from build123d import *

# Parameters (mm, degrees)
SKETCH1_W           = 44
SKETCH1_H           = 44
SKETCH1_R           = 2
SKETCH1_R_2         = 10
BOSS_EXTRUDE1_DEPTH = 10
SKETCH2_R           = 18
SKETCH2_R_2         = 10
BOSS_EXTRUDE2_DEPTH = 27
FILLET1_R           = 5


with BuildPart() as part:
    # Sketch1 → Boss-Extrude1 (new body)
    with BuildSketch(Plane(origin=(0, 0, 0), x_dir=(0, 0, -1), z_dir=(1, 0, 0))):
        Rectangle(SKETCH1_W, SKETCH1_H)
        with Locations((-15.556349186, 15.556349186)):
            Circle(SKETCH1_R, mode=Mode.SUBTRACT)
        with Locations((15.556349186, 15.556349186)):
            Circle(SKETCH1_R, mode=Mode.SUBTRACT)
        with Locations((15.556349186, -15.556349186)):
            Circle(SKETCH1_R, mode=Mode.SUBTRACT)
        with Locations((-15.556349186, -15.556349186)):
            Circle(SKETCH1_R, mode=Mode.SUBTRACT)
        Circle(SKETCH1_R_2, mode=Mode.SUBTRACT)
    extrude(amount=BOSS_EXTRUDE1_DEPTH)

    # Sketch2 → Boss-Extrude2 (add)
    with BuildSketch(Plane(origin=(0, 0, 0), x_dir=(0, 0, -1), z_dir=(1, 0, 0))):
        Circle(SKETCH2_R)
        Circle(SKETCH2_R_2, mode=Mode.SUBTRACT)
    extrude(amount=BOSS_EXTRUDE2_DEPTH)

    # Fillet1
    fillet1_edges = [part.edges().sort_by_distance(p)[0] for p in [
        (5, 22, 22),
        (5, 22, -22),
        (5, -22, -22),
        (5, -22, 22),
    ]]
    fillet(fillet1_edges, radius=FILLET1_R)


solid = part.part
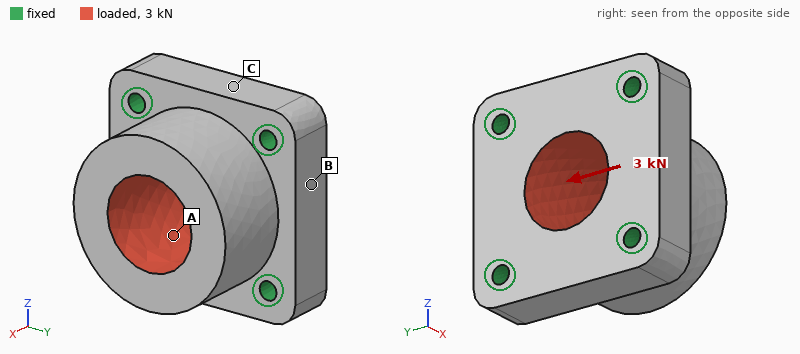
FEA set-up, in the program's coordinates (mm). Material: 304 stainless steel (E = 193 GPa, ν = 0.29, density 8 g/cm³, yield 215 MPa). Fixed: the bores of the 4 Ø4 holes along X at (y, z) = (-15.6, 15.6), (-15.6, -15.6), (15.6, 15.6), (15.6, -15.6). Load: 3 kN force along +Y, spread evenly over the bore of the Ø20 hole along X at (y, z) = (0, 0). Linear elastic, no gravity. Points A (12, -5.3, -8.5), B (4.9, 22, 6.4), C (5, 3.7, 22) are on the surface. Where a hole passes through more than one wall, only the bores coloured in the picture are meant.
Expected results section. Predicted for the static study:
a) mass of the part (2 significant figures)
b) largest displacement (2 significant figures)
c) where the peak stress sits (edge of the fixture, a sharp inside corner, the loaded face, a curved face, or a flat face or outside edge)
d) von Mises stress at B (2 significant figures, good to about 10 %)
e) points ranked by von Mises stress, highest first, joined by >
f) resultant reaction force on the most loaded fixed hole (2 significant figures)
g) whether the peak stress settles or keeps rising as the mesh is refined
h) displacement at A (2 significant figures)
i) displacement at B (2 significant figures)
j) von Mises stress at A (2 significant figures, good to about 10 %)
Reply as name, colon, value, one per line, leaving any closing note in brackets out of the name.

mass of the part: 220 g
largest displacement: 1.7 µm
where the peak stress sits: edge of the fixture
von Mises stress at B: 4.5 MPa
points ranked by von Mises stress, highest first, joined by >: A > B > C
resultant reaction force on the most loaded fixed hole: 870 N
whether the peak stress settles or keeps rising as the mesh is refined: keeps rising
displacement at A: 0.64 µm
displacement at B: 0.56 µm
von Mises stress at A: 6.6 MPa
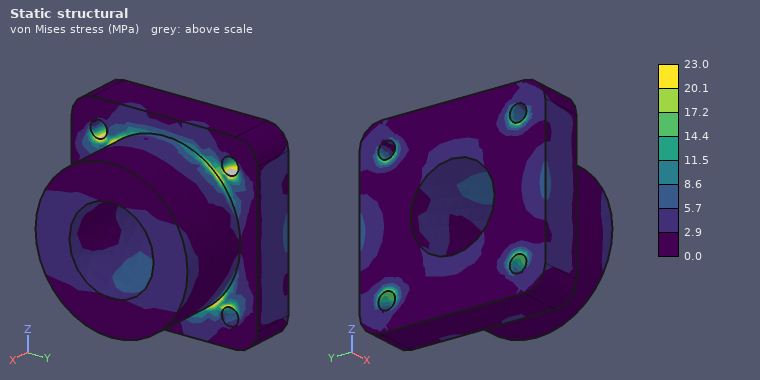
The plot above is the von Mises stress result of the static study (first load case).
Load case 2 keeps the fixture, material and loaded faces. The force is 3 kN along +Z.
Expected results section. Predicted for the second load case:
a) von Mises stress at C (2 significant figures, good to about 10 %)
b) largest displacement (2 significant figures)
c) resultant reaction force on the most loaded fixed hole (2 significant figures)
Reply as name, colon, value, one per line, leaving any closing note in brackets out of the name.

von Mises stress at C: 4.5 MPa
largest displacement: 1.7 µm
resultant reaction force on the most loaded fixed hole: 870 N
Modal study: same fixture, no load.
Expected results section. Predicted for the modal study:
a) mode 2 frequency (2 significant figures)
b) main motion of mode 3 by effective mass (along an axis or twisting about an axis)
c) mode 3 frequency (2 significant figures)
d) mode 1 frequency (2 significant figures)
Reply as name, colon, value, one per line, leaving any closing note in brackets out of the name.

mode 2 frequency: 20 kHz
main motion of mode 3 by effective mass: along X
mode 3 frequency: 25 kHz
mode 1 frequency: 20 kHz
